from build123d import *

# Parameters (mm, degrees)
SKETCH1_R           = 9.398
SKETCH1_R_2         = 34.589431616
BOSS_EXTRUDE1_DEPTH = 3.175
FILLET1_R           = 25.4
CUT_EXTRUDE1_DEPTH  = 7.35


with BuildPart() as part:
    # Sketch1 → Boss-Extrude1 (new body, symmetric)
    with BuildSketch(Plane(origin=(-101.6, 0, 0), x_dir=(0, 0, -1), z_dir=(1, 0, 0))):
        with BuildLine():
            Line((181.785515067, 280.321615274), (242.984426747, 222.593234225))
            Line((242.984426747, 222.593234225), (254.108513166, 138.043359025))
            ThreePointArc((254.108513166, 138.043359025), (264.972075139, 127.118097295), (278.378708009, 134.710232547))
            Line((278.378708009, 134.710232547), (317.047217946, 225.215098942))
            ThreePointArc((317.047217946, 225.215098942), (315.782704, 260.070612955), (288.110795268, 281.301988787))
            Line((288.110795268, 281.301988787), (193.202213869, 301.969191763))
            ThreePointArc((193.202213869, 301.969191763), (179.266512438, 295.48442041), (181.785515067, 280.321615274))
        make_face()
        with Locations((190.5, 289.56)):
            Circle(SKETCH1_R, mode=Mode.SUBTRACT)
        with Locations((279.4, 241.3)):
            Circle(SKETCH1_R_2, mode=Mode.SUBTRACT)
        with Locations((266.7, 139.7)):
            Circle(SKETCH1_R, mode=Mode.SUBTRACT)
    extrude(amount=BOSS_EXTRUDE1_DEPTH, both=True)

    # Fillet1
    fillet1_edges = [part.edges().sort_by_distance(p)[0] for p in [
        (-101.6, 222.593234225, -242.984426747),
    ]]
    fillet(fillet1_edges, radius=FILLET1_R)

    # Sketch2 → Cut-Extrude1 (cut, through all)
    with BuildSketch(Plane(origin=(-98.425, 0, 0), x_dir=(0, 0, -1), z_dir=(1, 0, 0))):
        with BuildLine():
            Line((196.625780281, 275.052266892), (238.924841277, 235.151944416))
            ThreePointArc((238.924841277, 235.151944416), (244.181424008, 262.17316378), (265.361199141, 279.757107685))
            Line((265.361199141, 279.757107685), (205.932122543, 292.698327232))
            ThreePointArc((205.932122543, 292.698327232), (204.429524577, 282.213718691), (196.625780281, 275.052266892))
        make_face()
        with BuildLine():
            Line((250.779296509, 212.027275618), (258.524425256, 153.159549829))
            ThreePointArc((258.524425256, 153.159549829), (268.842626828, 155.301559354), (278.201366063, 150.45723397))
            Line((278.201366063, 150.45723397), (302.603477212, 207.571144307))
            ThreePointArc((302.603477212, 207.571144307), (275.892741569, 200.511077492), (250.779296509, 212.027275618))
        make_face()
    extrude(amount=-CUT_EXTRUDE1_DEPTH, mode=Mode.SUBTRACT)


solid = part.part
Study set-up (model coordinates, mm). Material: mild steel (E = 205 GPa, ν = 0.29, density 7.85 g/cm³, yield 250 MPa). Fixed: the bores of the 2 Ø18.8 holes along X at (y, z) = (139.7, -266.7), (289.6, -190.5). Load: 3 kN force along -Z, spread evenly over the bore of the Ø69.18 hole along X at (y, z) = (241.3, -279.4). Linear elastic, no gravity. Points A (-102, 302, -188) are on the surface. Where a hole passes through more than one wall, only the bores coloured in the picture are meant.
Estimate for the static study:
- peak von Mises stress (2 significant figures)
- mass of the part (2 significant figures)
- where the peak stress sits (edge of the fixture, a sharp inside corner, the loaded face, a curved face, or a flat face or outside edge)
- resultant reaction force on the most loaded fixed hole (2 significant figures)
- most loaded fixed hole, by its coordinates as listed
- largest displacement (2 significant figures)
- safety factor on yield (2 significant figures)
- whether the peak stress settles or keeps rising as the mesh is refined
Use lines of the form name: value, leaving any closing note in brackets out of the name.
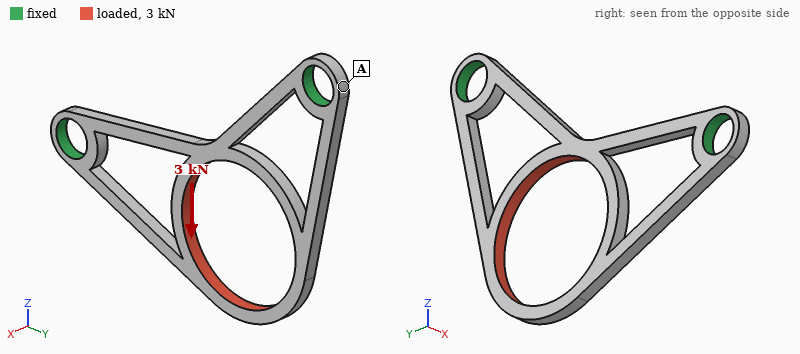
peak von Mises stress: 87 MPa
mass of the part: 200 g
where the peak stress sits: the loaded face
resultant reaction force on the most loaded fixed hole: 3.1 kN
most loaded fixed hole, by its coordinates as listed: (289.6, -190.5)
largest displacement: 68 µm
safety factor on yield: 2.9
whether the peak stress settles or keeps rising as the mesh is refined: settles
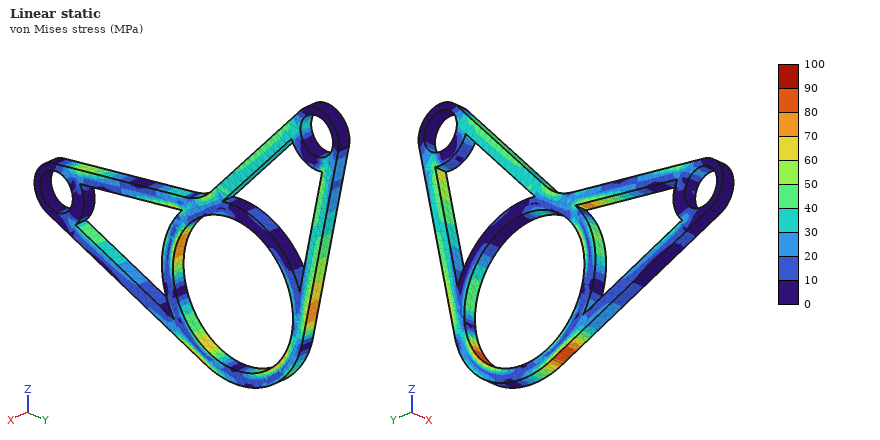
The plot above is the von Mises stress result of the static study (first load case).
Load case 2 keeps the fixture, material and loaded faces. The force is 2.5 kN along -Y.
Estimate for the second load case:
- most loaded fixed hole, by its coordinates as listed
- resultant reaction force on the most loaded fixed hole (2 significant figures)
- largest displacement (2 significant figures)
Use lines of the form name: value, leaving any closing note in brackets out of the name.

most loaded fixed hole, by its coordinates as listed: (139.7, -266.7)
resultant reaction force on the most loaded fixed hole: 2.3 kN
largest displacement: 69 µm
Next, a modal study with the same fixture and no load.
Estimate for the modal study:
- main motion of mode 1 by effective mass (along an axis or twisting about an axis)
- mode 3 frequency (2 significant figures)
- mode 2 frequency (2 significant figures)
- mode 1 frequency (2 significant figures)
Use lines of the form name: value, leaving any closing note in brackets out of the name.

main motion of mode 1 by effective mass: along X
mode 3 frequency: 1300 Hz
mode 2 frequency: 1300 Hz
mode 1 frequency: 440 Hz
